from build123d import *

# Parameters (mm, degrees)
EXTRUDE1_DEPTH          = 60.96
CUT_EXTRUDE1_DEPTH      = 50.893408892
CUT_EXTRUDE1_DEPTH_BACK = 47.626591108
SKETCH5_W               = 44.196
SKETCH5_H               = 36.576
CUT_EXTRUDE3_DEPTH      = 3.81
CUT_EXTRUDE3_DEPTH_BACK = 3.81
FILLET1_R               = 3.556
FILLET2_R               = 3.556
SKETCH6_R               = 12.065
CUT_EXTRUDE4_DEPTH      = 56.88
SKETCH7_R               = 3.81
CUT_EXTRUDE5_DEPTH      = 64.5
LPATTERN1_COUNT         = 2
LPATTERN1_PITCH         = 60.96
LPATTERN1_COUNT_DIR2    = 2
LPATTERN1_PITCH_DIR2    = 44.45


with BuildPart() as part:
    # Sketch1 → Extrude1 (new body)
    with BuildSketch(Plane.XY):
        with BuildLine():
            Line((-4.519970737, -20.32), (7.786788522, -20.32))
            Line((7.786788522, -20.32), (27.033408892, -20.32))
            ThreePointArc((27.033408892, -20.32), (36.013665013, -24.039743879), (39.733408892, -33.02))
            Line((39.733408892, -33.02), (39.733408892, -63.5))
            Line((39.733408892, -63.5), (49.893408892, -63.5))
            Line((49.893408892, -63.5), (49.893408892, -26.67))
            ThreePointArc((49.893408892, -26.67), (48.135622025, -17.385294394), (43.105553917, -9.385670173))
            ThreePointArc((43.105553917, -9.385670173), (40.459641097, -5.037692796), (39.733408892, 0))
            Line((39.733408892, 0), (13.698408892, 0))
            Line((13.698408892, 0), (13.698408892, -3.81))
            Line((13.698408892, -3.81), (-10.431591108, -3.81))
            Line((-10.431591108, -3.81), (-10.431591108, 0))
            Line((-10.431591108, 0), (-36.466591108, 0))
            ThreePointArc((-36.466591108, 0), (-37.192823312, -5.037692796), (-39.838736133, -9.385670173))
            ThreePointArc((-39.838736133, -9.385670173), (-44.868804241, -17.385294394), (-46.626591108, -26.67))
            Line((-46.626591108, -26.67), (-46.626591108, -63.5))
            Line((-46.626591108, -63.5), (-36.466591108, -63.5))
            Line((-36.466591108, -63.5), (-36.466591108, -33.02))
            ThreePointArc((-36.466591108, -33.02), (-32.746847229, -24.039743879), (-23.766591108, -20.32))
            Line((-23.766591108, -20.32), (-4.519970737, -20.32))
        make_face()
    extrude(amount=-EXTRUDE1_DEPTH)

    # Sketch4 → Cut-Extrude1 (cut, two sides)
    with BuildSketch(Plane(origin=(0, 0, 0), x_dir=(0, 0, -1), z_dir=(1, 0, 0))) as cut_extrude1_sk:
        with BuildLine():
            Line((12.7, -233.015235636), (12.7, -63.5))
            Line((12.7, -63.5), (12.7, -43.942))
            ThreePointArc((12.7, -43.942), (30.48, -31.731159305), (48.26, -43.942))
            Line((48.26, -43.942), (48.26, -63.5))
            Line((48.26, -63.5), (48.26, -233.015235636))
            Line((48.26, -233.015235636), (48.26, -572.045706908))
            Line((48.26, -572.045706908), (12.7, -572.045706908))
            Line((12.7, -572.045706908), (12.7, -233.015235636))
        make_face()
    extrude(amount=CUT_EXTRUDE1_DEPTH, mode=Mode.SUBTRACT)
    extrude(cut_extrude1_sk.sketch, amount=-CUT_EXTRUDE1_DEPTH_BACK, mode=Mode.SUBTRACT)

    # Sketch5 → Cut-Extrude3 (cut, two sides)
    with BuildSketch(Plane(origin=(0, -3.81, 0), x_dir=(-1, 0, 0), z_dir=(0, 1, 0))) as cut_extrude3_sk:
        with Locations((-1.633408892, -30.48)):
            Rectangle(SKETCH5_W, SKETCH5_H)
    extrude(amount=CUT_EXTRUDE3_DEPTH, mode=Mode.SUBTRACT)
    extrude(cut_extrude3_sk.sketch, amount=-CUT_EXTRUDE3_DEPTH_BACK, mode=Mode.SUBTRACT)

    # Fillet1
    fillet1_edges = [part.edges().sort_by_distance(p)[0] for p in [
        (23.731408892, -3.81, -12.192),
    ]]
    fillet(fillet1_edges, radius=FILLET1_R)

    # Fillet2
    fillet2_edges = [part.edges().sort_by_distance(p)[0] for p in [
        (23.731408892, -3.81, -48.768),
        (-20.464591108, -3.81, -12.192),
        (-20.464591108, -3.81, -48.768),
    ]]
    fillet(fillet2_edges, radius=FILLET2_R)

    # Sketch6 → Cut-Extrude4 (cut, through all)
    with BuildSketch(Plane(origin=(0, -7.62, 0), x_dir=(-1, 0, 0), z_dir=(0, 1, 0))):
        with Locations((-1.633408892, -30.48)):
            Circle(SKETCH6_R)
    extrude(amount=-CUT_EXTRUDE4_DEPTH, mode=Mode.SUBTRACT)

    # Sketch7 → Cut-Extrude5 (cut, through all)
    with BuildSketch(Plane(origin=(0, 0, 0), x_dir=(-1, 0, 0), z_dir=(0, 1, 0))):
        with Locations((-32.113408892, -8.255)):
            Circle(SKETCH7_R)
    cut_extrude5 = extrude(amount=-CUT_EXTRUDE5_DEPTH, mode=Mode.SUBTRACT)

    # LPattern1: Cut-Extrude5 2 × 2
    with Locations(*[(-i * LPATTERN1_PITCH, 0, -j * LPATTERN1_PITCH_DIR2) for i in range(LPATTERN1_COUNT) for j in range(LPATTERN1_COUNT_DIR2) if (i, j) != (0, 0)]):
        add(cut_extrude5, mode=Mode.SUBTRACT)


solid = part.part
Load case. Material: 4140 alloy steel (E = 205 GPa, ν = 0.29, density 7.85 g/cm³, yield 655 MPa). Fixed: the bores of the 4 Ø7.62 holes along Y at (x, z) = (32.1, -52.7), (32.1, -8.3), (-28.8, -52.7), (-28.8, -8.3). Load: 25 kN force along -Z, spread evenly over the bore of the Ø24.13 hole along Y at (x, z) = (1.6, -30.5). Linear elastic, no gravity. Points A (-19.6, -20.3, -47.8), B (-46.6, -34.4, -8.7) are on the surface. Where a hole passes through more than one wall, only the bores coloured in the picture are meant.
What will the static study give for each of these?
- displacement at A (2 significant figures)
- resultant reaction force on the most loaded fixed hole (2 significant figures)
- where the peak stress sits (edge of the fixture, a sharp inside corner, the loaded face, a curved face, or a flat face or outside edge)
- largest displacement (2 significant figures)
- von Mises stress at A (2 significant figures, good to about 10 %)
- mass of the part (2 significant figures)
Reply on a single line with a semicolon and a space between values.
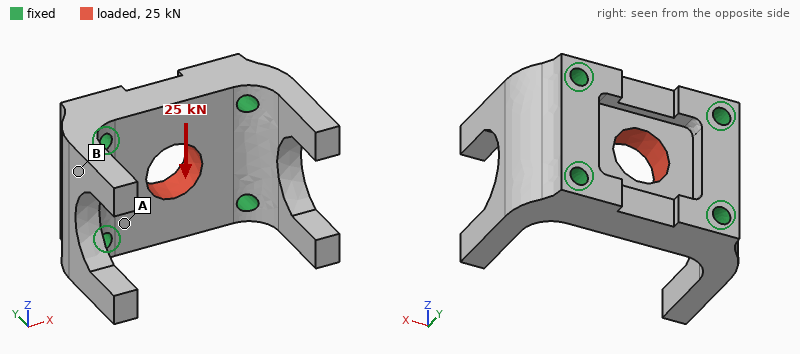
1.8 µm; 7.2 kN; edge of the fixture; 6.6 µm; 31 MPa; 920 g
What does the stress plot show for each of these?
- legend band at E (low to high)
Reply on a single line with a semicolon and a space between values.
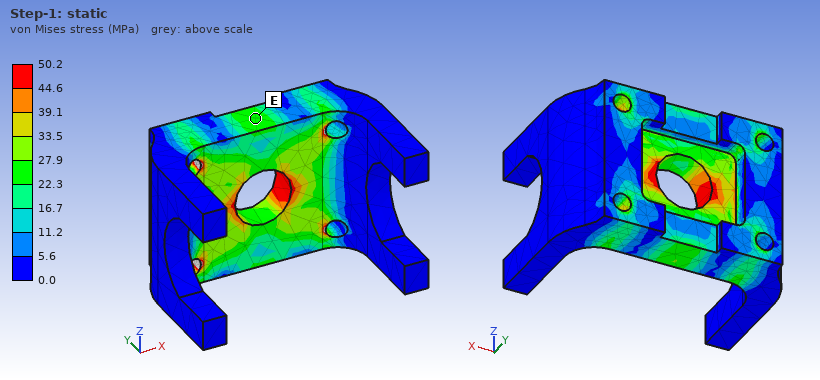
22.3 to 27.9 MPa
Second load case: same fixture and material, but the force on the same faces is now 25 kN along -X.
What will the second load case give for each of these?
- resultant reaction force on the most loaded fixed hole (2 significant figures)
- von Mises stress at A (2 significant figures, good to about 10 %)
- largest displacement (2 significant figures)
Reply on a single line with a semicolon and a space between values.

6.4 kN; 24 MPa; 3.3 µm
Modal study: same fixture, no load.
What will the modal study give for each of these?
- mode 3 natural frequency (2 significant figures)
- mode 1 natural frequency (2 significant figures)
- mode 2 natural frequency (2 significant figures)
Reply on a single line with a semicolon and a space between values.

5500 Hz; 5400 Hz; 5400 Hz
